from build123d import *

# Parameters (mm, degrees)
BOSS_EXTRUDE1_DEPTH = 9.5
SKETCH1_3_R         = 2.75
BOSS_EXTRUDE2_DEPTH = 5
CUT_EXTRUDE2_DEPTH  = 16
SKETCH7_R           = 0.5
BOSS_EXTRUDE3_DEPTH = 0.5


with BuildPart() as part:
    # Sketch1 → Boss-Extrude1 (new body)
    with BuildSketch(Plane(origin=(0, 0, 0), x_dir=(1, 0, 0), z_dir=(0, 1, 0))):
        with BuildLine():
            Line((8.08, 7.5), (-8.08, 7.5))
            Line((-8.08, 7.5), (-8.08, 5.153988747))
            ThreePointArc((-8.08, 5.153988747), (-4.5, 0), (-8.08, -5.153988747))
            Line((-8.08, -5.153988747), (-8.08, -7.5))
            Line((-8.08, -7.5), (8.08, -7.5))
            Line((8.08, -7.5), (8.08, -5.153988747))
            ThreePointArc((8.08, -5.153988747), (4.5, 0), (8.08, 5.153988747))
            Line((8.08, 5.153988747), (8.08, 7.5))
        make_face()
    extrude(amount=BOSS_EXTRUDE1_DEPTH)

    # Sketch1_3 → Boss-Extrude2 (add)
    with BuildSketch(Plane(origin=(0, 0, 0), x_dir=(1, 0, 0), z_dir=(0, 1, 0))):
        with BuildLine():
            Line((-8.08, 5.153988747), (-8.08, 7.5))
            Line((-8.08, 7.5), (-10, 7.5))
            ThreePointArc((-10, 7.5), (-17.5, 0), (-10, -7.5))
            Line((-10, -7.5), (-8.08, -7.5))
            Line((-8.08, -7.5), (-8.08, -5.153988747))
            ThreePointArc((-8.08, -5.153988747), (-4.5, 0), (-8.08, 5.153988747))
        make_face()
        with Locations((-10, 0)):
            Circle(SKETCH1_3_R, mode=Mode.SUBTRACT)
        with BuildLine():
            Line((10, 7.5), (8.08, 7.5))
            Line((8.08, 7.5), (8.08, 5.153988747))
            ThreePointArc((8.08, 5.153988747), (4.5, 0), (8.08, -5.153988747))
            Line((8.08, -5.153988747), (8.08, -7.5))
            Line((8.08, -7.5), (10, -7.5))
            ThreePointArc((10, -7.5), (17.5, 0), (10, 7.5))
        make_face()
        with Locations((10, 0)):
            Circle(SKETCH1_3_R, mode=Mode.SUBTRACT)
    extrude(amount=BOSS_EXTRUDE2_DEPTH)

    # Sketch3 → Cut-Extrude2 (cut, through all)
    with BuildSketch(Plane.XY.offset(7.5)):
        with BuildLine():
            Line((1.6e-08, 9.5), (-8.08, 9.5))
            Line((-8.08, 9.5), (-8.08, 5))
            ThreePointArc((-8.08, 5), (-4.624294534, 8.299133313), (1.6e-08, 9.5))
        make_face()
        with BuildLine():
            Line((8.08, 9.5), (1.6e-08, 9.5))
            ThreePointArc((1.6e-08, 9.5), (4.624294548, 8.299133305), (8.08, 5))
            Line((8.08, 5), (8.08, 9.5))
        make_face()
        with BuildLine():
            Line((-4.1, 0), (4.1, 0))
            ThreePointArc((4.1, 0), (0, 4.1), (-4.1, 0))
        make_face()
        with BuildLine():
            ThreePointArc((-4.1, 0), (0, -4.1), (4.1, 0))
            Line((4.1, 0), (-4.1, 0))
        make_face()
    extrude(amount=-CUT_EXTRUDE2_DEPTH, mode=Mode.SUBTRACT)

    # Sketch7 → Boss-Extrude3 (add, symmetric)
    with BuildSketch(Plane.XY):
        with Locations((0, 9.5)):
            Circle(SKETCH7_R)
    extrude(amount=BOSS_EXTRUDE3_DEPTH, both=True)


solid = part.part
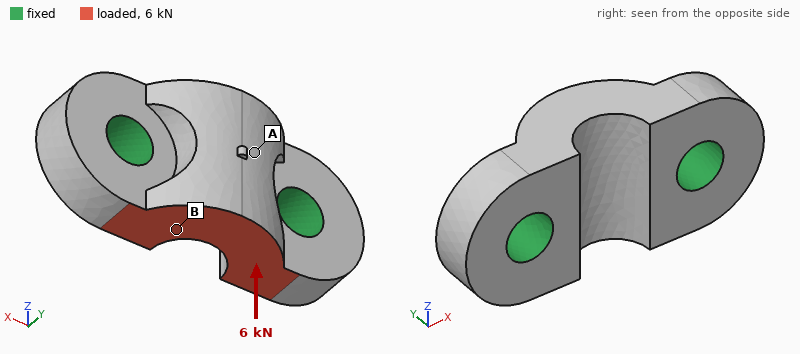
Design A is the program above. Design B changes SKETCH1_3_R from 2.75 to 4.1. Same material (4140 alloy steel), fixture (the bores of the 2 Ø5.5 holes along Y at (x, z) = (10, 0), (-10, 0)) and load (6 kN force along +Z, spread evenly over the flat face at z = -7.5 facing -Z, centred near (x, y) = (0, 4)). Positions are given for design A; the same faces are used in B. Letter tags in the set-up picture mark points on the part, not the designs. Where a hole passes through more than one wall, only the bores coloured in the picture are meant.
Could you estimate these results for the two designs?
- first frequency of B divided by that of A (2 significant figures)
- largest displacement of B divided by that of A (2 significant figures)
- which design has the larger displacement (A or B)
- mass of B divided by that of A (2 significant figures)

1.3
0.65
A
0.88
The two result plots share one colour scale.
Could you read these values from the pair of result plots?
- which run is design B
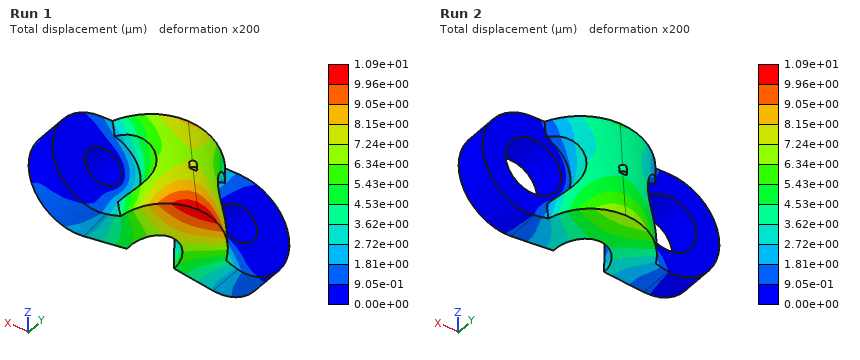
Run 2
